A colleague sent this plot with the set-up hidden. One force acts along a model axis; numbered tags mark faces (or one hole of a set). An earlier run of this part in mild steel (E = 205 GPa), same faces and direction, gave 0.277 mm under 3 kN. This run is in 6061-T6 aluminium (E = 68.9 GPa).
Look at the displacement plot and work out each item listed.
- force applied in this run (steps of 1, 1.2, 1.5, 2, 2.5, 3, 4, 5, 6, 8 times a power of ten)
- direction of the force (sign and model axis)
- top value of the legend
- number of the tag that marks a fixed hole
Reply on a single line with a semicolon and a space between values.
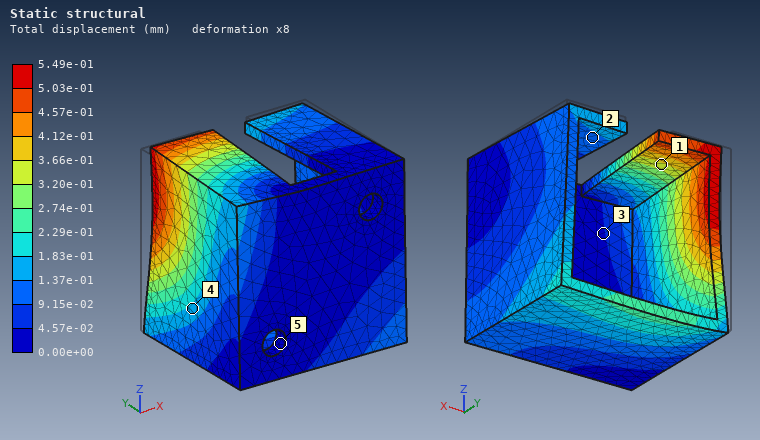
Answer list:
2 kN; +X; 5.49e-01 mm; 5
